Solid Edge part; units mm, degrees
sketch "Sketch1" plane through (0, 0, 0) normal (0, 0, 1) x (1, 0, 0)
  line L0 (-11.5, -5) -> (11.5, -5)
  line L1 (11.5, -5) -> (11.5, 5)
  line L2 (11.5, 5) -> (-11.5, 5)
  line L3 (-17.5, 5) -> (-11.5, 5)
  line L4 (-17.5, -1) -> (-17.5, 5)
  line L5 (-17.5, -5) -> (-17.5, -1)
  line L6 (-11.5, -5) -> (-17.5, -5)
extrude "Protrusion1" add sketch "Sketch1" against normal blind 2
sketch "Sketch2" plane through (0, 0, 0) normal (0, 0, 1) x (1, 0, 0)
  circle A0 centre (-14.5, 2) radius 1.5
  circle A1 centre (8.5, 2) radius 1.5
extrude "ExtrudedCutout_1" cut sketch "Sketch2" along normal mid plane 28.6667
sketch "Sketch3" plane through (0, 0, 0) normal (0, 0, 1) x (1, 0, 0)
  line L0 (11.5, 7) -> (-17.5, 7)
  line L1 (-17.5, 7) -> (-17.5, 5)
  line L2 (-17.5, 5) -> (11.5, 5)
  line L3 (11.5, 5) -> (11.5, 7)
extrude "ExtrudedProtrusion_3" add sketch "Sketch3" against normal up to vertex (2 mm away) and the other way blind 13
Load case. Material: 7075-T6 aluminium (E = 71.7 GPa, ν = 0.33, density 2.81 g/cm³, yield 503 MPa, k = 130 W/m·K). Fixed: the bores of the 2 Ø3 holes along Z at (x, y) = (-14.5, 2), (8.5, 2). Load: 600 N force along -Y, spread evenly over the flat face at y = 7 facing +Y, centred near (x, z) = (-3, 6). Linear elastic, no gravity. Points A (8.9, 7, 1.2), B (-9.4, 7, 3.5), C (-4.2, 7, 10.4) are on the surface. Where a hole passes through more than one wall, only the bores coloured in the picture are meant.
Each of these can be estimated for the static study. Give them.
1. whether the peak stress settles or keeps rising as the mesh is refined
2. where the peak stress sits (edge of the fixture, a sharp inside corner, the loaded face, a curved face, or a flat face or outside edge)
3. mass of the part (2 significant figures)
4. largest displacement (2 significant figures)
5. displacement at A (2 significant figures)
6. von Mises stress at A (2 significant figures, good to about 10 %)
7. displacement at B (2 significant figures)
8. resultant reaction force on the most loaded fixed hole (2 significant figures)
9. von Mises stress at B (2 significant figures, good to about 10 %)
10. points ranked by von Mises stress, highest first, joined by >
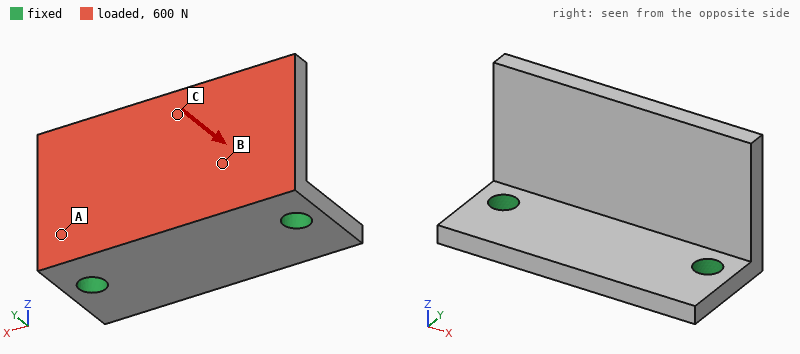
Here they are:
keeps rising
edge of the fixture
4.0 g
0.27 mm
0.043 mm
150 MPa
0.079 mm
300 N
82 MPa
A > B > C
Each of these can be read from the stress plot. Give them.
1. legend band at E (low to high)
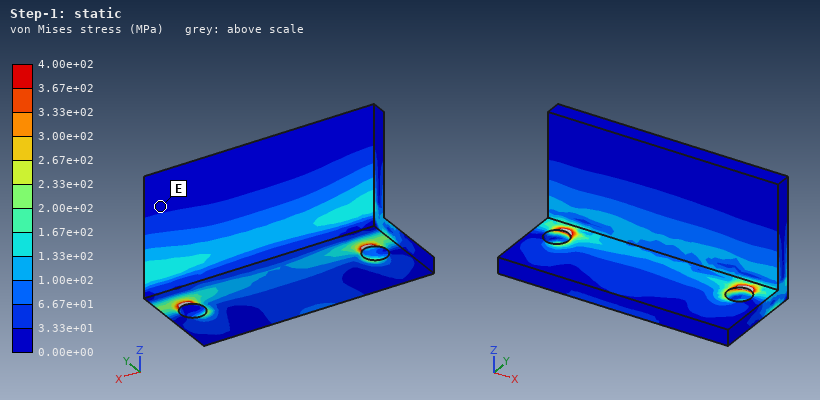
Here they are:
0.00e+00 to 3.33e+01 MPa
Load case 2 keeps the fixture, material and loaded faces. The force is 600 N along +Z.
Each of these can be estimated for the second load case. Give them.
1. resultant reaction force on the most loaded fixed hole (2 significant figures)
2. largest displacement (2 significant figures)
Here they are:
310 N
95 µm
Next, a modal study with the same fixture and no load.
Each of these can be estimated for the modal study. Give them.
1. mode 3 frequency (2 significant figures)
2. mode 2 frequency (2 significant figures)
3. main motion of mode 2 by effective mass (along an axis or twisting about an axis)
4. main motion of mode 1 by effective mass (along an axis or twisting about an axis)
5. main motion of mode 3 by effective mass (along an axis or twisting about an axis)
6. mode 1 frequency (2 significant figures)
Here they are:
20 kHz
10 kHz
twisting about Z
along Y
along Z
5900 Hz
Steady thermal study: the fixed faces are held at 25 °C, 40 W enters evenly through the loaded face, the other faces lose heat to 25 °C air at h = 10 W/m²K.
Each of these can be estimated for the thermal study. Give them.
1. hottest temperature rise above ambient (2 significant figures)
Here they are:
62 K
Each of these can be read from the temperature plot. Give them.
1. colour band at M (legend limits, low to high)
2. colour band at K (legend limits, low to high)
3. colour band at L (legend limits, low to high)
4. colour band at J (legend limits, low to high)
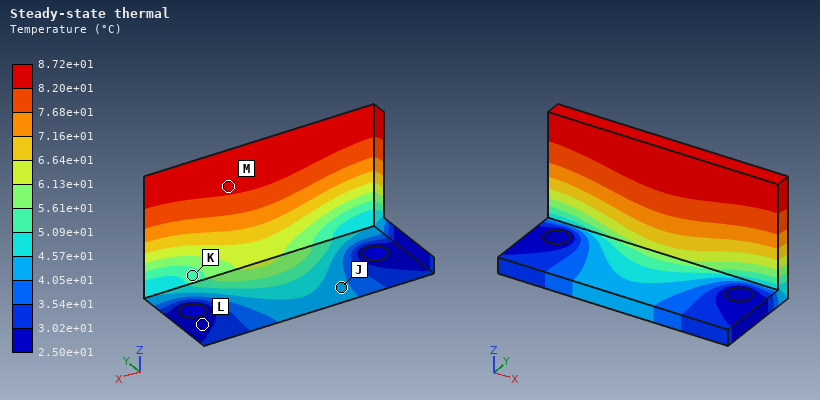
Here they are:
8.20e+01 to 8.72e+01 °C
5.09e+01 to 5.61e+01 °C
2.50e+01 to 3.02e+01 °C
4.05e+01 to 4.57e+01 °C
